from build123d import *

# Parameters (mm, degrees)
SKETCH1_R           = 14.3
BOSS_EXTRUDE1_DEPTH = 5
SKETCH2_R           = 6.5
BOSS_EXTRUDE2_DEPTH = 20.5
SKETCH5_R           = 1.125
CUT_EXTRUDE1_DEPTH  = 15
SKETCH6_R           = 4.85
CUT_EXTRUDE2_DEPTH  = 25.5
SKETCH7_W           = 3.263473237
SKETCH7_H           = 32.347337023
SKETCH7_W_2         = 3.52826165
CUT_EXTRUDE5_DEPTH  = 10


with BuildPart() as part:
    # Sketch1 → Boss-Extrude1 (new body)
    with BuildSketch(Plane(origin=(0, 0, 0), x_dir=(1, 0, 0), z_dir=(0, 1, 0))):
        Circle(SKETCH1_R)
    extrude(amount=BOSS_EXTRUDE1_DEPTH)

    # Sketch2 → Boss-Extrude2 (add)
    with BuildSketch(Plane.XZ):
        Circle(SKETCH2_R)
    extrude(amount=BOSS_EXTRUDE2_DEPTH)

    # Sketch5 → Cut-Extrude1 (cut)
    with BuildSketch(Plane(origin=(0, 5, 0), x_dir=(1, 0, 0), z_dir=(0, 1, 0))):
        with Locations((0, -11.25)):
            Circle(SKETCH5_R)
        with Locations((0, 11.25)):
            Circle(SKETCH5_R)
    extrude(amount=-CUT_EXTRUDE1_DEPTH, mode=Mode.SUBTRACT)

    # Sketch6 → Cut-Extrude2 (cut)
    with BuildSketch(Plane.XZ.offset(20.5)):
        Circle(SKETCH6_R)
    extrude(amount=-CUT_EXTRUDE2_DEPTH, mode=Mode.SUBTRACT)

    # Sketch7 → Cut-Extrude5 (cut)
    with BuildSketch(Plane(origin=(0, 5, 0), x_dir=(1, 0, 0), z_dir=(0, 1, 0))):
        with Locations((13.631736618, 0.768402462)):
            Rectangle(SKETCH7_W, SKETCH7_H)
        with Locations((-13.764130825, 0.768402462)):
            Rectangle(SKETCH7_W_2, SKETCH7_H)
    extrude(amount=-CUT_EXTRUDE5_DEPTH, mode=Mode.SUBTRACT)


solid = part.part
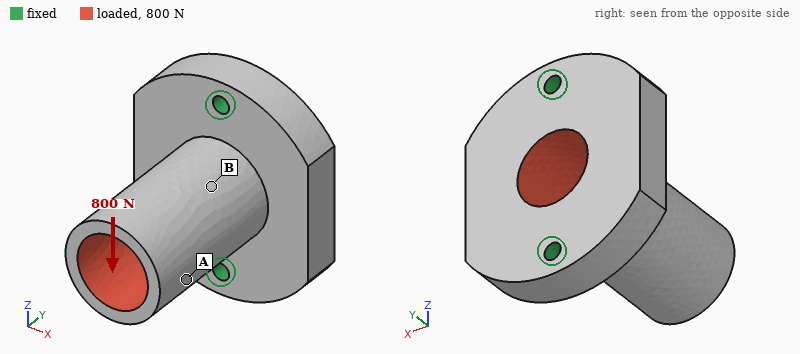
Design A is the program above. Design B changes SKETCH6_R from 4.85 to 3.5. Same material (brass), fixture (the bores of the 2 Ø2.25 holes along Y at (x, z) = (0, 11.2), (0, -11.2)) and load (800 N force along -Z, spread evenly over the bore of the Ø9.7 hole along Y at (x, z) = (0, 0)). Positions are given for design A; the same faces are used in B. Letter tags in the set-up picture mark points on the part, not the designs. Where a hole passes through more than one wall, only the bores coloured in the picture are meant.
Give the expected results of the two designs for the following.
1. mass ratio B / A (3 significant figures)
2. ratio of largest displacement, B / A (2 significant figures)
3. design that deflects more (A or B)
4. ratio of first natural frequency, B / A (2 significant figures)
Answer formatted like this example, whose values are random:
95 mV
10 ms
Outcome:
1.24
0.75
A
0.87
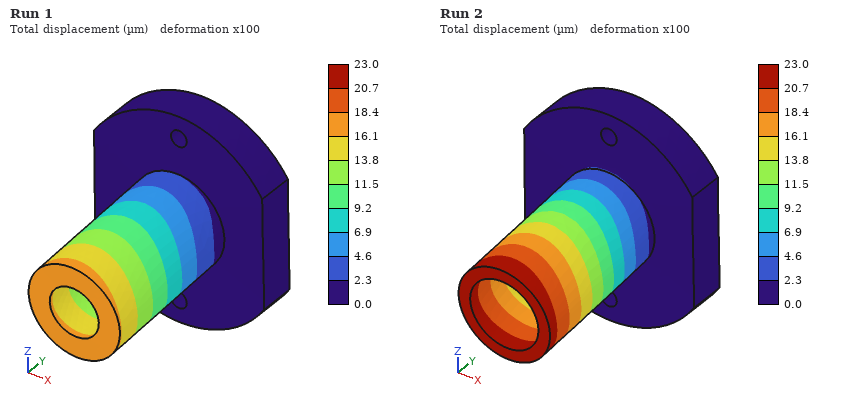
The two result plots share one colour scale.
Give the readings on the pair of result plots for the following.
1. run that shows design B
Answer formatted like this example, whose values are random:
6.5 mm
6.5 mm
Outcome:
Run 1
